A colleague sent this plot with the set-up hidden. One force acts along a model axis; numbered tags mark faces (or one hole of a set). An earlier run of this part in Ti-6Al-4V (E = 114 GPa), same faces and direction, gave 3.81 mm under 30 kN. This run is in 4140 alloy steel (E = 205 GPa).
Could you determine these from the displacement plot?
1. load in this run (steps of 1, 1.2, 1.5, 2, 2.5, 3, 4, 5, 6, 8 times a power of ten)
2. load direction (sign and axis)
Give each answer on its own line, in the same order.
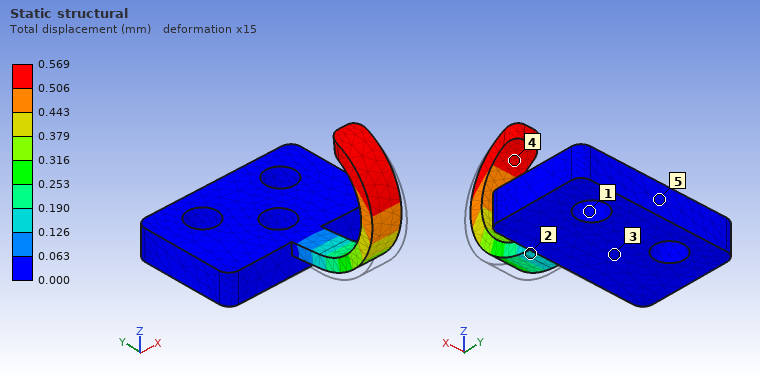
8 kN
+Z
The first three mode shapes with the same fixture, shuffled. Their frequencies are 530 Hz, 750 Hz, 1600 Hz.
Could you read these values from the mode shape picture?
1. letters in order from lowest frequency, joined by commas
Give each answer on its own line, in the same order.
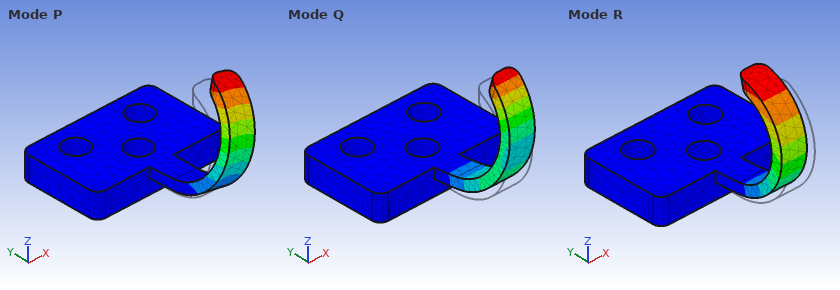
R, P, Q
